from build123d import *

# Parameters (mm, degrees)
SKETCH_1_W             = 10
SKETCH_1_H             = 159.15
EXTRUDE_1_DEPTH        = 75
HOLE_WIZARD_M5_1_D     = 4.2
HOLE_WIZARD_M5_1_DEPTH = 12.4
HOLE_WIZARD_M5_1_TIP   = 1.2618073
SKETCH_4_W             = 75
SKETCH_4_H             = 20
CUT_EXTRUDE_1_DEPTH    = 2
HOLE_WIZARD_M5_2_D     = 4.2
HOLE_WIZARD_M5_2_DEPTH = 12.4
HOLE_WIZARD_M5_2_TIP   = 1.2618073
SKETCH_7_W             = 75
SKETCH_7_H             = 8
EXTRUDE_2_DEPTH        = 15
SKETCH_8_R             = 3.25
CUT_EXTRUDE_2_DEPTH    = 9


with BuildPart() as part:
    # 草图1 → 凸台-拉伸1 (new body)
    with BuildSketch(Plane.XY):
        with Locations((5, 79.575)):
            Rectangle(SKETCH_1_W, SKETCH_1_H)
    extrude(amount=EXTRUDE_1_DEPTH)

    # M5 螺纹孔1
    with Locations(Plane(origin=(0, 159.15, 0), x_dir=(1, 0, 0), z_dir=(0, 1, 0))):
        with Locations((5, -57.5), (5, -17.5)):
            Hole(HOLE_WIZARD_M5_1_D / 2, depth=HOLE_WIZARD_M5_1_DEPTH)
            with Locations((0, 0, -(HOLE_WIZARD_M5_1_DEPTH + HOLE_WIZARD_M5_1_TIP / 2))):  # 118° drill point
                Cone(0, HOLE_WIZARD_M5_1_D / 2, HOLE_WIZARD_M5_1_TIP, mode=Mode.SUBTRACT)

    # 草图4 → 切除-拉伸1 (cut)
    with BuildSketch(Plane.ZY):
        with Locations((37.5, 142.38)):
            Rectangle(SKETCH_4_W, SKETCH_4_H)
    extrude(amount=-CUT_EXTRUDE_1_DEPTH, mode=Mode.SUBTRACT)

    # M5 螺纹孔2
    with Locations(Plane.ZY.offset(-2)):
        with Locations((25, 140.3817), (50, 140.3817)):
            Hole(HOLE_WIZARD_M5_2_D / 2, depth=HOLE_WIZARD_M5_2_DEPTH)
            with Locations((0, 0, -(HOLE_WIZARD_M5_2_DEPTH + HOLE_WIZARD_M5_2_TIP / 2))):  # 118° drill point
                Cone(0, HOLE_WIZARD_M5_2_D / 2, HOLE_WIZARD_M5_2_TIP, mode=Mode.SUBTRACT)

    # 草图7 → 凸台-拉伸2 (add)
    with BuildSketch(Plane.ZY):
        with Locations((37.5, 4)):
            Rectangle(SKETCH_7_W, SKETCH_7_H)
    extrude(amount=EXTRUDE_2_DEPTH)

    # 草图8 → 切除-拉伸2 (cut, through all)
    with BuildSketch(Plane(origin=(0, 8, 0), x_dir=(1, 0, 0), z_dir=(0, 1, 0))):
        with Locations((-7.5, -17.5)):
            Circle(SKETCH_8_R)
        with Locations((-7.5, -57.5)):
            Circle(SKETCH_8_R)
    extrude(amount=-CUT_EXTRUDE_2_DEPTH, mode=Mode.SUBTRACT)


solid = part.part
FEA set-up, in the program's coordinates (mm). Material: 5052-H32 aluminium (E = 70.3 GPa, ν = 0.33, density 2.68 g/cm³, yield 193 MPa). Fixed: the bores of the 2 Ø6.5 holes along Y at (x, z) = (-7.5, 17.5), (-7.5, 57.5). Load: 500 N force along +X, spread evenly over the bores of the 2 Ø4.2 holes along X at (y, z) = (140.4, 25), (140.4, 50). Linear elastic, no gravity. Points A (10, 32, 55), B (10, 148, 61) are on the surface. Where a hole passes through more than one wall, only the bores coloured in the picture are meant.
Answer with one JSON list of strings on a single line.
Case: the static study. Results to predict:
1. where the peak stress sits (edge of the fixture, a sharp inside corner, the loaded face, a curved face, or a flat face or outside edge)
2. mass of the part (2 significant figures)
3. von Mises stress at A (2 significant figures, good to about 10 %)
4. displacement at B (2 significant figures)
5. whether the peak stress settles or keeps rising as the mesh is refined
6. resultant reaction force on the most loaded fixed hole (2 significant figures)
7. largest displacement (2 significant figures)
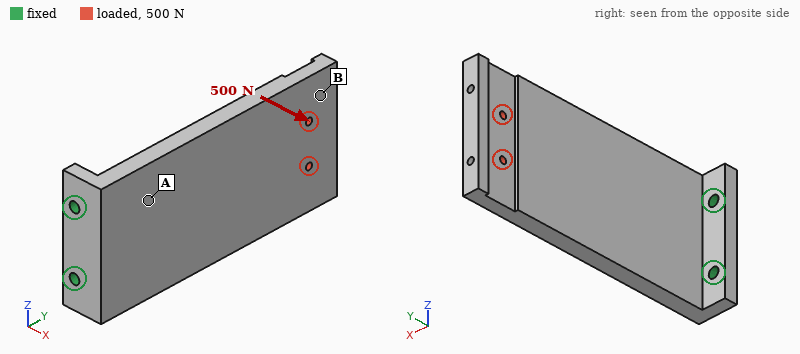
["edge of the fixture", "330 g", "41 MPa", "1.5 mm", "keeps rising", "430 N", "1.7 mm"]
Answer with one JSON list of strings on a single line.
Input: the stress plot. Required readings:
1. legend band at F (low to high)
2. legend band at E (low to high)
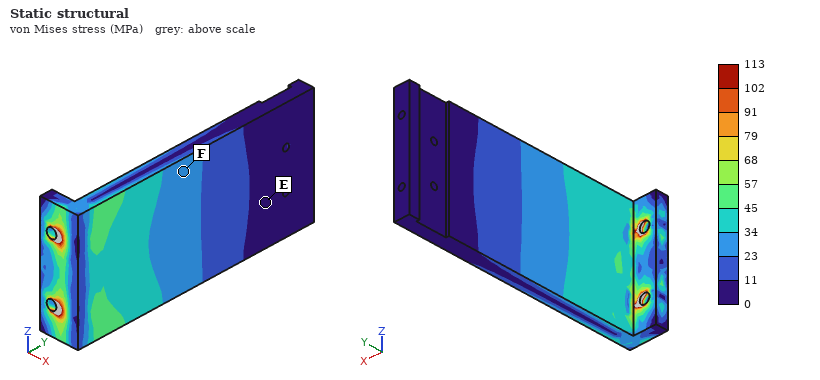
["23 to 34 MPa", "0 to 11 MPa"]
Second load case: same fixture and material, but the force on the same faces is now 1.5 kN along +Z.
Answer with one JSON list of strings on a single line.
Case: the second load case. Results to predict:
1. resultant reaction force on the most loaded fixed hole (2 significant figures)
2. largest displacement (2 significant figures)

["4.6 kN", "0.27 mm"]
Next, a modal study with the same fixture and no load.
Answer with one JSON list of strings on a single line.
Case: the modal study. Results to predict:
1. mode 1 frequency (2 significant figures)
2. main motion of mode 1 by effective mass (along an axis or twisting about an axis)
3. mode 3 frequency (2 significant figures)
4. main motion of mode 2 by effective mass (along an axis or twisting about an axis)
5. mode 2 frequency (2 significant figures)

["290 Hz", "along X", "1500 Hz", "along Z", "1100 Hz"]
